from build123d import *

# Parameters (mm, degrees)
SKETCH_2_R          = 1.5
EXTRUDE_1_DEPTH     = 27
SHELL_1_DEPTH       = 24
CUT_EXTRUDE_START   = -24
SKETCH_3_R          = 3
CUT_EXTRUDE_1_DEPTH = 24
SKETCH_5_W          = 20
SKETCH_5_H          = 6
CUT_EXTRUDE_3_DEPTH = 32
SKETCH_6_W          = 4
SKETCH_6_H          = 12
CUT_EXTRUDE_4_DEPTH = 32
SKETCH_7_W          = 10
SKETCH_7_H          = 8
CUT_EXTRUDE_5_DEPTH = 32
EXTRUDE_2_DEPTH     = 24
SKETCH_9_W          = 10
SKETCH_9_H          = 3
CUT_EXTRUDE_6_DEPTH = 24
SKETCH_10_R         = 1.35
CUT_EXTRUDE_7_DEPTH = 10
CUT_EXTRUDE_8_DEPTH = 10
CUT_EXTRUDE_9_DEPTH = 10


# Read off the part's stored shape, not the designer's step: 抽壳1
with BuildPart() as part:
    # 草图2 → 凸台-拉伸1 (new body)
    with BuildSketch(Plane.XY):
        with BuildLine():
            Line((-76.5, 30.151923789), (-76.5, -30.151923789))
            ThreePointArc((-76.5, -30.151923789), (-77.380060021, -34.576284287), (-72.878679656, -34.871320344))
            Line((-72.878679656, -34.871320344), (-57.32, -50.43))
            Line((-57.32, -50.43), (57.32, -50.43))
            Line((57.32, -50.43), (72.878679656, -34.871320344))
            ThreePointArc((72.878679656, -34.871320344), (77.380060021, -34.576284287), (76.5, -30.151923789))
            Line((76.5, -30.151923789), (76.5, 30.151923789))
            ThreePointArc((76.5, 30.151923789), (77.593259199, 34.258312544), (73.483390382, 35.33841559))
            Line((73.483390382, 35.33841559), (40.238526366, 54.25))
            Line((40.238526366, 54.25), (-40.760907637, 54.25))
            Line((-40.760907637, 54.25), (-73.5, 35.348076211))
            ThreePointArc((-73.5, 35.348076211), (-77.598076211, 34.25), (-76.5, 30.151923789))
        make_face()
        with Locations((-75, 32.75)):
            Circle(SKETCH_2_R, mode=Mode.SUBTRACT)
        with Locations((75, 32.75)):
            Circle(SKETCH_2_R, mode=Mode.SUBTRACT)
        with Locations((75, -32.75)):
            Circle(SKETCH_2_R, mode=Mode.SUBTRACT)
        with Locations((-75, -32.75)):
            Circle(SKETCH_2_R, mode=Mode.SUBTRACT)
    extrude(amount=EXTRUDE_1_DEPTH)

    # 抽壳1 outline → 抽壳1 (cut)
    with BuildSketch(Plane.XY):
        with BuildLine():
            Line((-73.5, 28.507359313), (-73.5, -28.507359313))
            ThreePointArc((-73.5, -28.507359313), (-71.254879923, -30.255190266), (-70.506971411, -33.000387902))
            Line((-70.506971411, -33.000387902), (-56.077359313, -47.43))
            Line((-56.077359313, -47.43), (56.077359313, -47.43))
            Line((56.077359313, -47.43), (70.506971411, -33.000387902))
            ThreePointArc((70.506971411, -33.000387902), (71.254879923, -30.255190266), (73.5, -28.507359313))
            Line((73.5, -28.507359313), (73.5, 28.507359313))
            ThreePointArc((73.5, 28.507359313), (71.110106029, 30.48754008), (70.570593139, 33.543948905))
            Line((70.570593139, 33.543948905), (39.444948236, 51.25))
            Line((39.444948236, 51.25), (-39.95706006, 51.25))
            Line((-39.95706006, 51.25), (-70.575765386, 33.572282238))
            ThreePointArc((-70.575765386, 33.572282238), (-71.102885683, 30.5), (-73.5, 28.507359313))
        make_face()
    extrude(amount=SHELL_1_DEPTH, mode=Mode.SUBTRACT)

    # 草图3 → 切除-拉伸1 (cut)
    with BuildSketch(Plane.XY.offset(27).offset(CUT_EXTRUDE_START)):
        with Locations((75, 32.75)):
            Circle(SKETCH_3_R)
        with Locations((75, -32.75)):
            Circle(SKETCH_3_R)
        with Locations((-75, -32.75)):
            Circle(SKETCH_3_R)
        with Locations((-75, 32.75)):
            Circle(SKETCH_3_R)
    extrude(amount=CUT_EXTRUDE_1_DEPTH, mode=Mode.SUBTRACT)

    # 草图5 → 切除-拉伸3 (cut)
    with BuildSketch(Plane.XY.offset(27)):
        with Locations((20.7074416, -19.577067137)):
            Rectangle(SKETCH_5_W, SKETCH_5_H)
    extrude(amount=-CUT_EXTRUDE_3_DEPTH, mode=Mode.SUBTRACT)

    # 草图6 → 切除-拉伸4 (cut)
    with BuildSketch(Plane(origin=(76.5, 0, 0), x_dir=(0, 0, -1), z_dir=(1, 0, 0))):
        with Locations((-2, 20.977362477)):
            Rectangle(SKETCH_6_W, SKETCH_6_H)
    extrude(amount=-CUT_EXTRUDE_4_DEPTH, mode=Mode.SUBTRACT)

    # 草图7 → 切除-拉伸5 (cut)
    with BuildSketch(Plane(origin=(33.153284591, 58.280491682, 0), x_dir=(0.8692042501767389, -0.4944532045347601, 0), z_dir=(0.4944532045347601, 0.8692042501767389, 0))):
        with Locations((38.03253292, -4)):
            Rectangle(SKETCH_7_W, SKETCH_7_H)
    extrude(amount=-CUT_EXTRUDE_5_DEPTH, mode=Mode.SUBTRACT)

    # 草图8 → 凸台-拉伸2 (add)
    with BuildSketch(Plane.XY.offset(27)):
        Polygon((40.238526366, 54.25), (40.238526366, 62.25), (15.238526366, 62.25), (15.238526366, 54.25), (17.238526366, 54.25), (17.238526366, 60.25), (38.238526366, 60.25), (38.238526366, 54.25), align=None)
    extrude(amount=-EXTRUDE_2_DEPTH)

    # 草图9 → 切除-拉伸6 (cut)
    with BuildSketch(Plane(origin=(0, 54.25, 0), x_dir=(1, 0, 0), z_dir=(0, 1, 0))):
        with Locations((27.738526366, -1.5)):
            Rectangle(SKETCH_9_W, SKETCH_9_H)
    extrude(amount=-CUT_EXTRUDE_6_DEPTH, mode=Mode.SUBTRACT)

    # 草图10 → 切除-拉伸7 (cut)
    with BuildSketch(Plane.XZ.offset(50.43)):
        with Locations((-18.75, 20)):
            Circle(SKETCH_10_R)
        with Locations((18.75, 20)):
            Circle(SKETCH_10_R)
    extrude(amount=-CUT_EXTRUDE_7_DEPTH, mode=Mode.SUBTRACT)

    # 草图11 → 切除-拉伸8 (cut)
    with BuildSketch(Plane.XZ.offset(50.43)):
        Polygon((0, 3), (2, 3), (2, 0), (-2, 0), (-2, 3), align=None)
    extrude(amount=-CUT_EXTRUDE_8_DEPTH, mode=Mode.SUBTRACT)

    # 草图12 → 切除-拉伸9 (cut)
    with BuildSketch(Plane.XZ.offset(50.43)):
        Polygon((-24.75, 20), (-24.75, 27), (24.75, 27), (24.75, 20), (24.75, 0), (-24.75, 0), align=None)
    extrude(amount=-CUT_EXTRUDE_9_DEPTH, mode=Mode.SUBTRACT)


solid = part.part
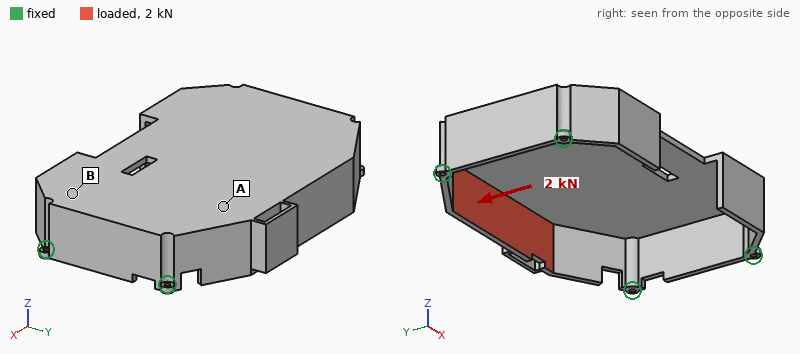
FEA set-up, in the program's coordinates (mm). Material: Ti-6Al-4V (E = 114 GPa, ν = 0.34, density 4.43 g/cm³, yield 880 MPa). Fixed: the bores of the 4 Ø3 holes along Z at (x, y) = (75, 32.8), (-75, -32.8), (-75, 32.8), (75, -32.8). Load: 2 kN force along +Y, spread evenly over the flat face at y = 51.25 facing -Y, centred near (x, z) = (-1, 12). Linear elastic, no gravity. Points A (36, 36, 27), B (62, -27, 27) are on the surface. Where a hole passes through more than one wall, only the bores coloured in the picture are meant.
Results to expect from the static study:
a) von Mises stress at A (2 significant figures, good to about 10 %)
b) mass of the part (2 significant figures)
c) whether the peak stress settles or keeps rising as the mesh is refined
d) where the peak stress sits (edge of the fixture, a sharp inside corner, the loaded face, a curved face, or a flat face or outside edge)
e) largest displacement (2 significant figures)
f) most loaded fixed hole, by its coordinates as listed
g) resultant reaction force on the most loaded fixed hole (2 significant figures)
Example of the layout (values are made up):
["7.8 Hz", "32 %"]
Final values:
["21 MPa", "320 g", "keeps rising", "edge of the fixture", "0.27 mm", "(-75, 32.8)", "1.1 kN"]
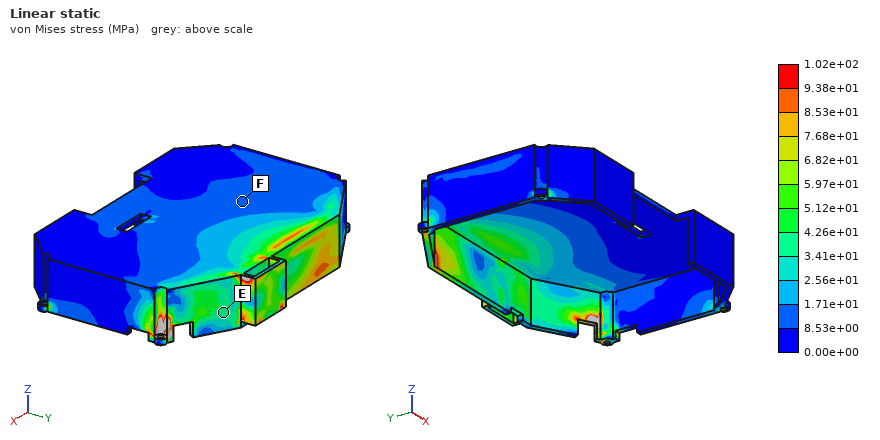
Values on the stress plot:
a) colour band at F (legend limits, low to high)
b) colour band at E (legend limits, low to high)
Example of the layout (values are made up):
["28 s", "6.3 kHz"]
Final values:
["8.53e+00 to 1.71e+01 MPa", "3.41e+01 to 4.26e+01 MPa"]
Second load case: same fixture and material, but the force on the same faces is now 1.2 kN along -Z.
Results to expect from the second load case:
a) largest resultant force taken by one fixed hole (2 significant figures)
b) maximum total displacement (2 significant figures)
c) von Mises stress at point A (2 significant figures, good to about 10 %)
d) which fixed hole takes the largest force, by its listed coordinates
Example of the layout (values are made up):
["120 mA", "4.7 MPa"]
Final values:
["1.1 kN", "88 µm", "11 MPa", "(-75, 32.8)"]
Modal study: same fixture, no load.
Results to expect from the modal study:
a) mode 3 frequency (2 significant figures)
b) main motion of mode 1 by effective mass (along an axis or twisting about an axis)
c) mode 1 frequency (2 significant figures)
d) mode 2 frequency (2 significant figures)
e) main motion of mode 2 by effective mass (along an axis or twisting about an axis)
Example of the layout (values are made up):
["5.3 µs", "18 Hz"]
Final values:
["2200 Hz", "along Z", "1100 Hz", "1500 Hz", "along X"]
